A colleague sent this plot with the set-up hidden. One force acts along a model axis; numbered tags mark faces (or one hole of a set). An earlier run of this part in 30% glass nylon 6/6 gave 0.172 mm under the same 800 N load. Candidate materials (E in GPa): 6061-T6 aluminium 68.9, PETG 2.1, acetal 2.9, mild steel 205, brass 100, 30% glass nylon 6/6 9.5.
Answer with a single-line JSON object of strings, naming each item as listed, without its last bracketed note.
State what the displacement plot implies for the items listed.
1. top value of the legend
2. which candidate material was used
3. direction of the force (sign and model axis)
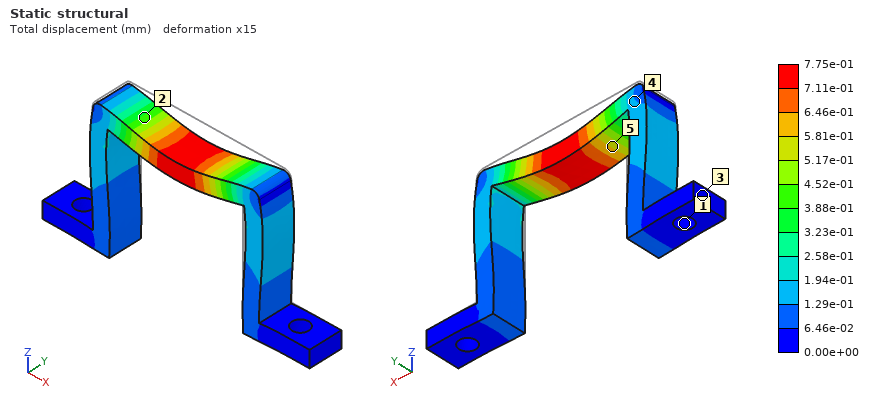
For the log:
{"top value of the legend": "7.75e-01 mm", "which candidate material was used": "PETG", "direction of the force": "-Z"}
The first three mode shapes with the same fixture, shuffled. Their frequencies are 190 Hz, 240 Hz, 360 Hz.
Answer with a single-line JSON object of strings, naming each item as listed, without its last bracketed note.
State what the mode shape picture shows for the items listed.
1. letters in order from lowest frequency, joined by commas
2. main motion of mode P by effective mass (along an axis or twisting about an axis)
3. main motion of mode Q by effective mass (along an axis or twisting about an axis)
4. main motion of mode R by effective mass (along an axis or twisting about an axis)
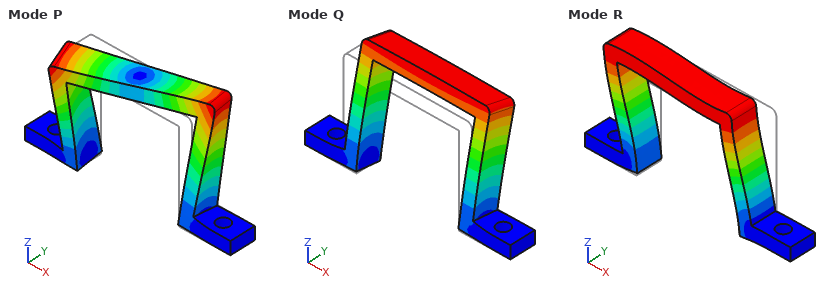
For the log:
{"letters in order from lowest frequency, joined by commas": "Q, R, P", "main motion of mode P by effective mass": "twisting about Z", "main motion of mode Q by effective mass": "along Y", "main motion of mode R by effective mass": "along X"}
